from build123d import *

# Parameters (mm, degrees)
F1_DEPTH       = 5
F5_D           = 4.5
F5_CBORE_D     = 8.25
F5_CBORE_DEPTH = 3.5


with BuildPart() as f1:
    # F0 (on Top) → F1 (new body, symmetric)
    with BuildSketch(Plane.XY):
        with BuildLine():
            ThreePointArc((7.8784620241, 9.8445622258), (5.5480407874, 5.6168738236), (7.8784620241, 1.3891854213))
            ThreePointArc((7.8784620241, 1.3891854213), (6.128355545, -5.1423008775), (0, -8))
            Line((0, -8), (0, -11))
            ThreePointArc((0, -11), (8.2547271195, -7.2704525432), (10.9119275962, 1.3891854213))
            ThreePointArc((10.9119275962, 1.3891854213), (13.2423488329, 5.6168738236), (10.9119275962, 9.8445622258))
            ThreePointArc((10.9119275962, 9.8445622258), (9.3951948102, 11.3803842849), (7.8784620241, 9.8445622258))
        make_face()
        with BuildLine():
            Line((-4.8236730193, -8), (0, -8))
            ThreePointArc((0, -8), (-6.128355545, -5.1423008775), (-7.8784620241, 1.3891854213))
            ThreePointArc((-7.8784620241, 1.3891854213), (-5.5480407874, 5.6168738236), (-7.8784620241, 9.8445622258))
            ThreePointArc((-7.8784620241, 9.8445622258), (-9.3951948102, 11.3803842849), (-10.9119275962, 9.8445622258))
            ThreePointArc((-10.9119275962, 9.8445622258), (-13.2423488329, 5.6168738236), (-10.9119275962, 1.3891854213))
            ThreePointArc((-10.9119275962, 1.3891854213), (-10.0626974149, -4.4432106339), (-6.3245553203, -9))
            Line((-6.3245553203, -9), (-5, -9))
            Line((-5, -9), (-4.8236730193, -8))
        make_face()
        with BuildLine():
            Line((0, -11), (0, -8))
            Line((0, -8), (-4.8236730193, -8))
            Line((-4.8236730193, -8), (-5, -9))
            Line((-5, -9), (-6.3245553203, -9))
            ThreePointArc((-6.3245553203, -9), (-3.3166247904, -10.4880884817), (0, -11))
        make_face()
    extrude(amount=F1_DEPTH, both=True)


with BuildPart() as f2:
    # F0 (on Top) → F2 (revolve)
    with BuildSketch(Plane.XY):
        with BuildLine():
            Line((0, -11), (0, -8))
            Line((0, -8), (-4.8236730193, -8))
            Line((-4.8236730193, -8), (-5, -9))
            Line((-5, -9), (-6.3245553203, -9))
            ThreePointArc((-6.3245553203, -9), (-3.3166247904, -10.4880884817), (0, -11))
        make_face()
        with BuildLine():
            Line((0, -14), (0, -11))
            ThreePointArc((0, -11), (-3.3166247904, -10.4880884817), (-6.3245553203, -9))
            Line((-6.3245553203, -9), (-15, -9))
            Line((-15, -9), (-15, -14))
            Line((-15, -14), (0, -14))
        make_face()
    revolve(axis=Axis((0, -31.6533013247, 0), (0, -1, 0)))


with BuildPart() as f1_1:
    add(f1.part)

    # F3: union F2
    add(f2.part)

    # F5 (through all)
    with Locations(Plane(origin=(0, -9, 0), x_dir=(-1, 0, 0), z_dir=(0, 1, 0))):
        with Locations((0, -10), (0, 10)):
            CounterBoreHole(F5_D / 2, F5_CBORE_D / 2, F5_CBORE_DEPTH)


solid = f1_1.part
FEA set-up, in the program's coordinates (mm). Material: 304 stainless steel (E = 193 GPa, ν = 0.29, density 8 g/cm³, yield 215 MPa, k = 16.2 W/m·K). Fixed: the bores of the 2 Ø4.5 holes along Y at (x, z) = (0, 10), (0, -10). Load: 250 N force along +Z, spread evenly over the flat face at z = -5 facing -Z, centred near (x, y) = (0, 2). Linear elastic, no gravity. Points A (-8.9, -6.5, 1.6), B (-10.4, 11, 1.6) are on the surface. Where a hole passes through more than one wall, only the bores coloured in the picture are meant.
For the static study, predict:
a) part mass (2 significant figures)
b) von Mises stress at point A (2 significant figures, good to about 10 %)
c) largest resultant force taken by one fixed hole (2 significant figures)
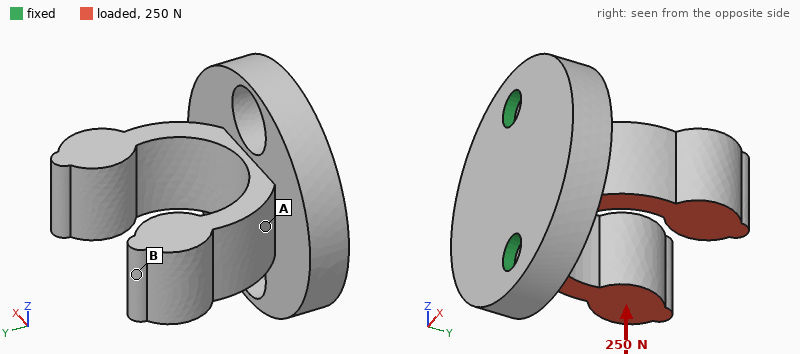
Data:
40 g
12 MPa
240 N
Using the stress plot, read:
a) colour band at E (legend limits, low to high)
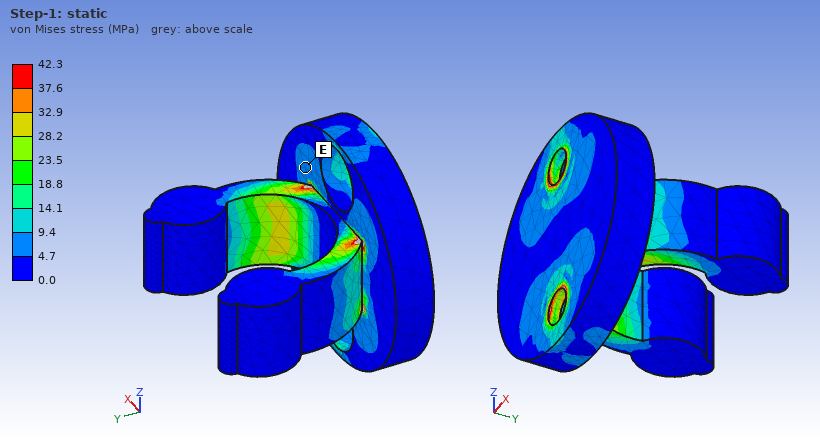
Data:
4.7 to 9.4 MPa
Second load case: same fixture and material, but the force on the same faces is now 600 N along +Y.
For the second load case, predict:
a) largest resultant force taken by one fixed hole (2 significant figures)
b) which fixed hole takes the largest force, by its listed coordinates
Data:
500 N
(0, -10)
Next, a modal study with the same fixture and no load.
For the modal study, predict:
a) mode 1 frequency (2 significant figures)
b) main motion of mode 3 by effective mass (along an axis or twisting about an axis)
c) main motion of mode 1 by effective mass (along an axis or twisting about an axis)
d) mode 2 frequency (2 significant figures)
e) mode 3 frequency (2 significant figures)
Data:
2900 Hz
along Z
along X
3900 Hz
7500 Hz
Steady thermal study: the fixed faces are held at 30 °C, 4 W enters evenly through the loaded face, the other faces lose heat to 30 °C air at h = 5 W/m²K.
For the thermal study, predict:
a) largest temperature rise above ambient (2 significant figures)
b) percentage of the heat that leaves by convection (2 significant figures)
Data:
63 K
9.8 %
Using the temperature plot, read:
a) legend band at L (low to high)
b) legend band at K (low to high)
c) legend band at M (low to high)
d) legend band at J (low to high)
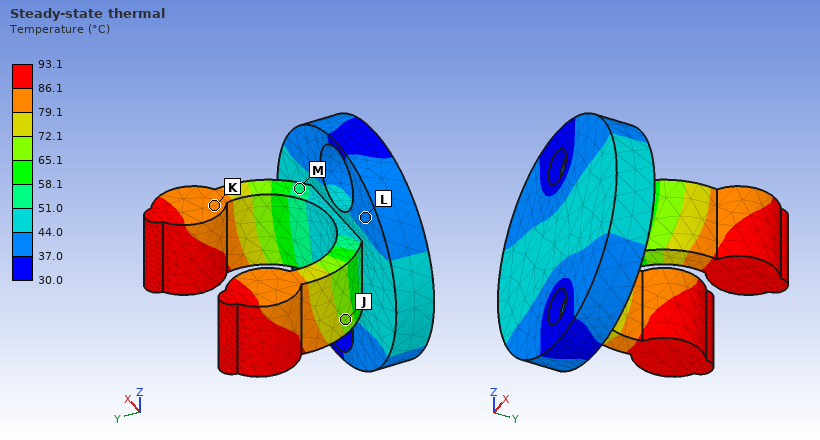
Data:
37.0 to 44.0 °C
79.1 to 86.1 °C
51.0 to 58.1 °C
65.1 to 72.1 °C
